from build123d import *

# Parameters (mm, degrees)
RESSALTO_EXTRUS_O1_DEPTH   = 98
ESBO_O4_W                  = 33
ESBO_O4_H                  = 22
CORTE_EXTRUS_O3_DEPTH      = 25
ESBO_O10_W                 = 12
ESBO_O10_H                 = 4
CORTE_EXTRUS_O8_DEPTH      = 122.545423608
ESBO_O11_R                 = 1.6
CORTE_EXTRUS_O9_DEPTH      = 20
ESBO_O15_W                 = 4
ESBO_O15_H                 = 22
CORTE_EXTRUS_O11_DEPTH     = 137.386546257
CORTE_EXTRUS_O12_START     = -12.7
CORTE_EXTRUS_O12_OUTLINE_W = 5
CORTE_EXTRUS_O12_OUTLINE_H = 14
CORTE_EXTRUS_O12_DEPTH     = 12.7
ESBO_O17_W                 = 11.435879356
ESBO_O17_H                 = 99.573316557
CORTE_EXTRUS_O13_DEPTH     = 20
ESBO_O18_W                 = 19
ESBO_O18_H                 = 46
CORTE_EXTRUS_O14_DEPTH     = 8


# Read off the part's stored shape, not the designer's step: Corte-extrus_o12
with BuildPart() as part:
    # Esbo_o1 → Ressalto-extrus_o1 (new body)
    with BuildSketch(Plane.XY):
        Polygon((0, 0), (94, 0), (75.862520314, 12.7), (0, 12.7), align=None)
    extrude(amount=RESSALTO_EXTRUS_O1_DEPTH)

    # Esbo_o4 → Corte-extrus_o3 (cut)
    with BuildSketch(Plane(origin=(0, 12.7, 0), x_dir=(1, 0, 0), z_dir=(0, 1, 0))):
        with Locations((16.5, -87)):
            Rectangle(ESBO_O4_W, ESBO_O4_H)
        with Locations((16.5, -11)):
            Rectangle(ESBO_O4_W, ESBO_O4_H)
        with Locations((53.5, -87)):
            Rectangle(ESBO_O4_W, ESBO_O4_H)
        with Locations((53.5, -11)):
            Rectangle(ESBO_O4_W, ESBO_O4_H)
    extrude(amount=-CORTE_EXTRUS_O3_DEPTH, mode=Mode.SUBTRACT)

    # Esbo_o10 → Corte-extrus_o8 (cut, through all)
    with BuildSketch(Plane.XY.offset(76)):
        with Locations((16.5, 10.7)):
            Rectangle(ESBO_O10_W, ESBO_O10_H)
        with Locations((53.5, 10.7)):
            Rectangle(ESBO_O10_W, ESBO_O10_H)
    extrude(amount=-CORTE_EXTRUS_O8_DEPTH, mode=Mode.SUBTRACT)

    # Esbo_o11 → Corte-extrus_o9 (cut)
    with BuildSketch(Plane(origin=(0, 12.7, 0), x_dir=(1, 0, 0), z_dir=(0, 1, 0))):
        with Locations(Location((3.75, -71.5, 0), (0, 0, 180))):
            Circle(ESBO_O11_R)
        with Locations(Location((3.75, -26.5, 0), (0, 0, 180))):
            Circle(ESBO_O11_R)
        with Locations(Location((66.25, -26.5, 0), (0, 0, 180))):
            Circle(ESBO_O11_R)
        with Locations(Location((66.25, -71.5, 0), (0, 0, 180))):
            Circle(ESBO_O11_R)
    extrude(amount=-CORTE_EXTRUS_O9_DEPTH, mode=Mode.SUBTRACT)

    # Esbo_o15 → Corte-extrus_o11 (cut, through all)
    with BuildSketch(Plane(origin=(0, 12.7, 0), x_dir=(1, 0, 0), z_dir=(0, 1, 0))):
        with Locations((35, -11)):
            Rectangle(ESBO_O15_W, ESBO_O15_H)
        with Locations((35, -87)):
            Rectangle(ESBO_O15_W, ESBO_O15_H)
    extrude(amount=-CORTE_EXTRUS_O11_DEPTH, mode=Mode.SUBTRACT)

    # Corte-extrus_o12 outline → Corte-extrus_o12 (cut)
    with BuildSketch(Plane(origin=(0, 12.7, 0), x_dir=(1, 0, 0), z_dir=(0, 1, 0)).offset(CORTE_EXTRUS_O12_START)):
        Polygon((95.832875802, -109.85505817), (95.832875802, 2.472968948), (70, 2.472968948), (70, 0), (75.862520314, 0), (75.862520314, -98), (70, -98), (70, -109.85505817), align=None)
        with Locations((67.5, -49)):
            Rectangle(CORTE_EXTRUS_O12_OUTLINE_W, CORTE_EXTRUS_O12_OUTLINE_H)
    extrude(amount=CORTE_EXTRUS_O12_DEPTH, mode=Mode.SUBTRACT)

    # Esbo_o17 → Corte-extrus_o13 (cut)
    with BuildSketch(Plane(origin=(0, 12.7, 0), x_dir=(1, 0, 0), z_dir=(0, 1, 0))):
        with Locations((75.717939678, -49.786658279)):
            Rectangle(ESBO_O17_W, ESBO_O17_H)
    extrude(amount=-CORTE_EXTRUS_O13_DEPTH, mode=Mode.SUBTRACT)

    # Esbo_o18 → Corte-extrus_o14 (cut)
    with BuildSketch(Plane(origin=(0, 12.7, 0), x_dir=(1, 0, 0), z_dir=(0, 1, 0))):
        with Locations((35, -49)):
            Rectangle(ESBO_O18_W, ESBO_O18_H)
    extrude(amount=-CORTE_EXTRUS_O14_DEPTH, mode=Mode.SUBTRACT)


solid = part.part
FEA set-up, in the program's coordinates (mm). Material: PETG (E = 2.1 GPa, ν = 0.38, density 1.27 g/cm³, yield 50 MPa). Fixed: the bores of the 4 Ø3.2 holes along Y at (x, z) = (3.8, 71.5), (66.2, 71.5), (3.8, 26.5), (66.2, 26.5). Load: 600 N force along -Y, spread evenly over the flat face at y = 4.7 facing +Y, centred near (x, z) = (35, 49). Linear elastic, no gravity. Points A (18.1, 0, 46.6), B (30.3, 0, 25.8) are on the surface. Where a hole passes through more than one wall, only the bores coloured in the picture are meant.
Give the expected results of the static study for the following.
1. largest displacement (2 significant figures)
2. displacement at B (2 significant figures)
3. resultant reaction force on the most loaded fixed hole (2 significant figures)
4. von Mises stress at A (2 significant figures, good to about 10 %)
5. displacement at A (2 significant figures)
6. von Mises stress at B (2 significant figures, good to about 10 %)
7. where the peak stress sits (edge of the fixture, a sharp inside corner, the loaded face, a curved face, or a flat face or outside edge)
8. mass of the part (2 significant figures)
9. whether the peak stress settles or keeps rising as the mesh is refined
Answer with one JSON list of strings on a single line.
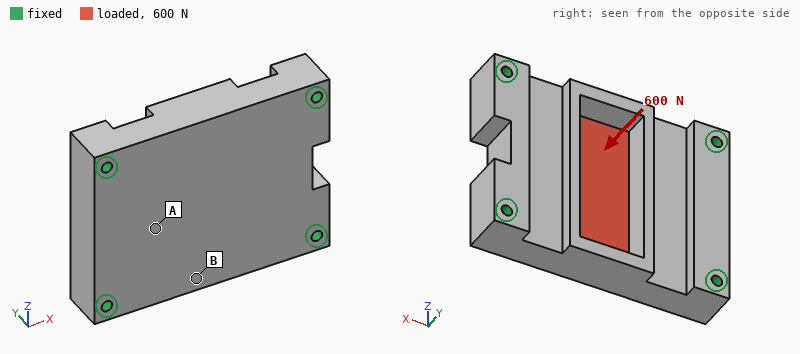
["0.23 mm", "0.14 mm", "220 N", "1.8 MPa", "0.11 mm", "4.5 MPa", "edge of the fixture", "44 g", "keeps rising"]
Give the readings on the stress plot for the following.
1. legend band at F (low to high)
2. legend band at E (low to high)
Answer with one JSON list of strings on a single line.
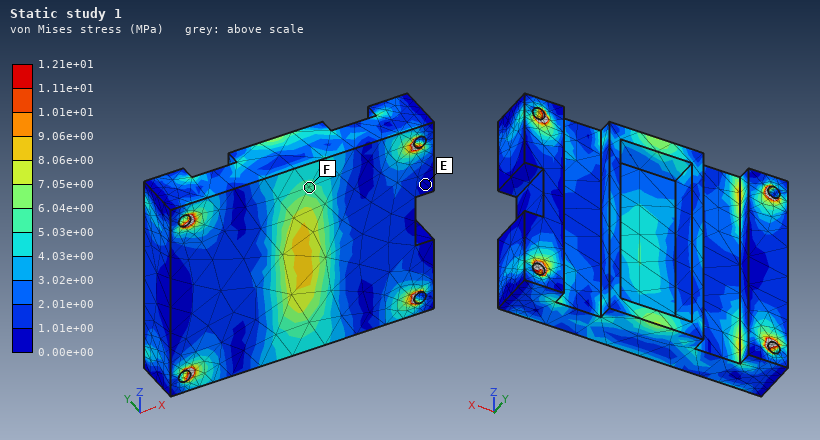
["5.03e+00 to 6.04e+00 MPa", "0.00e+00 to 1.01e+00 MPa"]
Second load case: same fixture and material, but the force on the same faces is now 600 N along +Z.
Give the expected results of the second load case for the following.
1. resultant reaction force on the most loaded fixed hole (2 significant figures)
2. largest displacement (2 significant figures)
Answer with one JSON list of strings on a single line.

["180 N", "39 µm"]
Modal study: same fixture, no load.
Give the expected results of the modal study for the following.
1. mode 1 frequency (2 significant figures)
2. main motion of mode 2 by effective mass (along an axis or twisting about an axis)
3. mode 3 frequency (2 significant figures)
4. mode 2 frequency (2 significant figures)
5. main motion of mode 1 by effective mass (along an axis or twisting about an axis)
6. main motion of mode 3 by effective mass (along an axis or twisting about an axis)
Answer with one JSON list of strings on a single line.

["2400 Hz", "twisting about X", "4300 Hz", "3400 Hz", "along Y", "twisting about Z"]
